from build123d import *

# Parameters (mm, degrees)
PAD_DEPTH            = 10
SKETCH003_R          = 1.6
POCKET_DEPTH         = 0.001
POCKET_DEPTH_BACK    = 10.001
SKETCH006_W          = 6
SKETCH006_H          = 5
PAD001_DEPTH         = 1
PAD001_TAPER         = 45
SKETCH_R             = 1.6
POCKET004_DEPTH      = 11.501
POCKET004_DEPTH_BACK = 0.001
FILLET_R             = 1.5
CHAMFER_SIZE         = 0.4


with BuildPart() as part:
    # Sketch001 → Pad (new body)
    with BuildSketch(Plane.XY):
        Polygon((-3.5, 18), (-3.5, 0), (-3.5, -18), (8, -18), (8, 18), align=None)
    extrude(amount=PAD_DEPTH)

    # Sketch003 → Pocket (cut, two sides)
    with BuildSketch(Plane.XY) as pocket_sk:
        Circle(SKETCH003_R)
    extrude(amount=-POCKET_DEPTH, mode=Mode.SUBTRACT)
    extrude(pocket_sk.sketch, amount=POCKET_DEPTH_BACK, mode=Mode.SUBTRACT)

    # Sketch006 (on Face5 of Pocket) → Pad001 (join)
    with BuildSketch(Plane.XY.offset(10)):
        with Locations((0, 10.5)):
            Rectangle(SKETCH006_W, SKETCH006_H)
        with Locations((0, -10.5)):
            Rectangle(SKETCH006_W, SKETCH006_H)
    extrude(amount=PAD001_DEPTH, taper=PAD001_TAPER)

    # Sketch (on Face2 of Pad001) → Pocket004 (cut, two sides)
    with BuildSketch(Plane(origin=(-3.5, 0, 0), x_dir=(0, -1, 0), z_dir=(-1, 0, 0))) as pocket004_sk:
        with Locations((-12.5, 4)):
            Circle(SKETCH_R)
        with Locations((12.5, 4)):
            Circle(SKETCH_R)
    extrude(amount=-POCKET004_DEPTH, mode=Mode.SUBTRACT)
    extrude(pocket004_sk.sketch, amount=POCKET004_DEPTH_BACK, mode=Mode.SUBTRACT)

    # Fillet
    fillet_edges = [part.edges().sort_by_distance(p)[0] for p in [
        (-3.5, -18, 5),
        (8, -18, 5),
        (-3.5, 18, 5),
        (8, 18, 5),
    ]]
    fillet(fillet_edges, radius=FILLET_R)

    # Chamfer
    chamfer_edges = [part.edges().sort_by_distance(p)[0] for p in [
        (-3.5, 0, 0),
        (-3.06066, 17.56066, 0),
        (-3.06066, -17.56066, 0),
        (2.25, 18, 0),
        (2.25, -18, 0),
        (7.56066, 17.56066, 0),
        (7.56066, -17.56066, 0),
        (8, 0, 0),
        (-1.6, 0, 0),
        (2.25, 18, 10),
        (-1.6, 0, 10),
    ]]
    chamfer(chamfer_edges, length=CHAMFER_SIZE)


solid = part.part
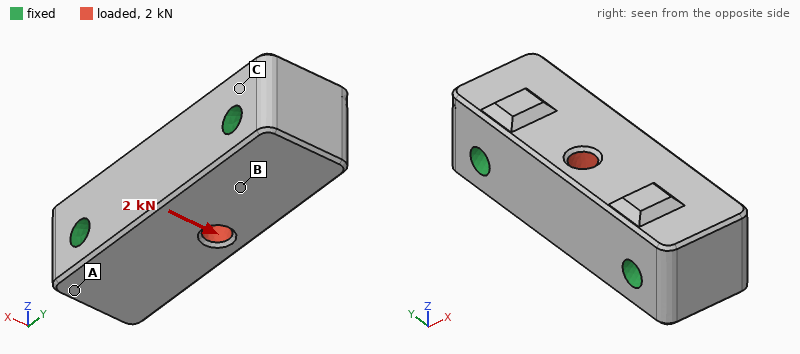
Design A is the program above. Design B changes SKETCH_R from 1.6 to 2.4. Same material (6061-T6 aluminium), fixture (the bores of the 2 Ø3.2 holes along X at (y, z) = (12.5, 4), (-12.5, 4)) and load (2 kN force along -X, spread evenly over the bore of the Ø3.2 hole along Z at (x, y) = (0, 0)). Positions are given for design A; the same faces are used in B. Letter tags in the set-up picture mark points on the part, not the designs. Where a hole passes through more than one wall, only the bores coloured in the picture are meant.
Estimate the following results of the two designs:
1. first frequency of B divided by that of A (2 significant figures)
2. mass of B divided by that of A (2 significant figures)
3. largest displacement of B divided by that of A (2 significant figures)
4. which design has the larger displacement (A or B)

1.2
0.94
0.88
A
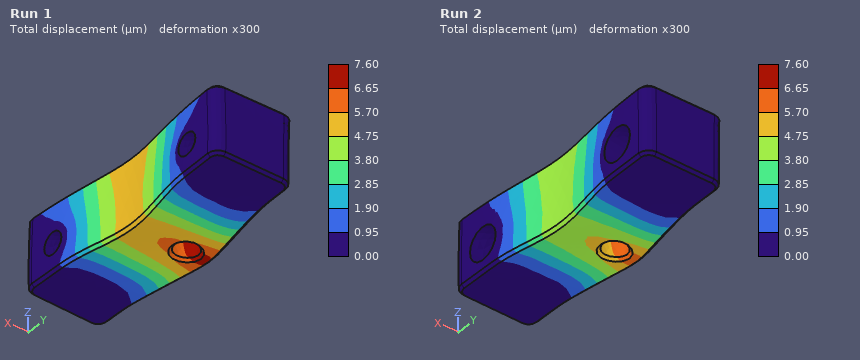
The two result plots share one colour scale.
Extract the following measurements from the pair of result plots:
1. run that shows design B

Run 2
